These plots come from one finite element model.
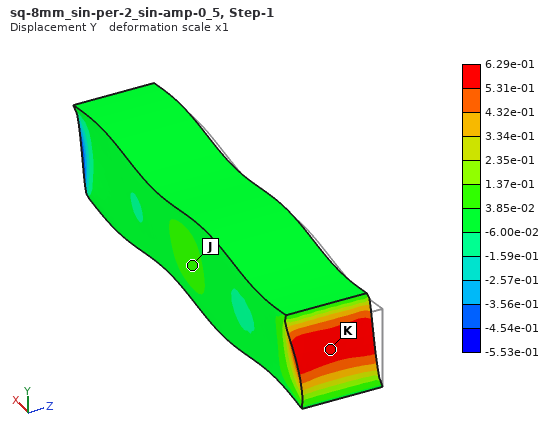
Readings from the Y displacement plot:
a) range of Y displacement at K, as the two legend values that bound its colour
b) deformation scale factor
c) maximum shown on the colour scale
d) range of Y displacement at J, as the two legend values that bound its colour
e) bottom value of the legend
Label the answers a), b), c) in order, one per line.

a) 5.31e-01 to 6.29e-01
b) 1
c) 6.29e-01
d) 3.85e-02 to 1.37e-01
e) -5.53e-01
